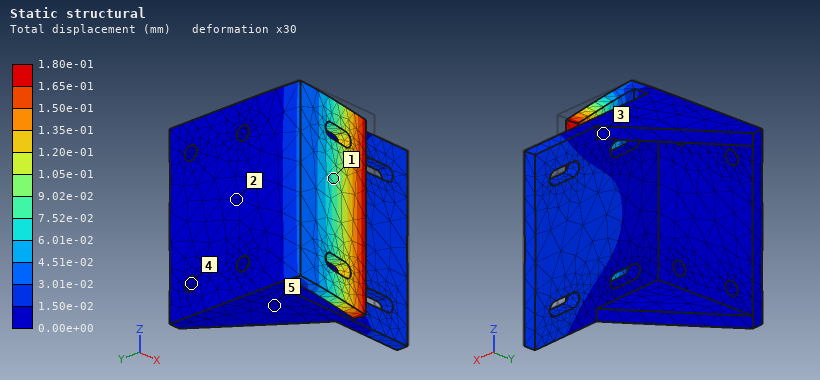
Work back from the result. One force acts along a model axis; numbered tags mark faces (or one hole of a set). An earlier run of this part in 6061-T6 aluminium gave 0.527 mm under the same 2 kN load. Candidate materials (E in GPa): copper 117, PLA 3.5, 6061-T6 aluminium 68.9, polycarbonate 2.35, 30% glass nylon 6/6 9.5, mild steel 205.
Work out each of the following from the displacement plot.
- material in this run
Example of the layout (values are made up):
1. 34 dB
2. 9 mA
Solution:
1. mild steel
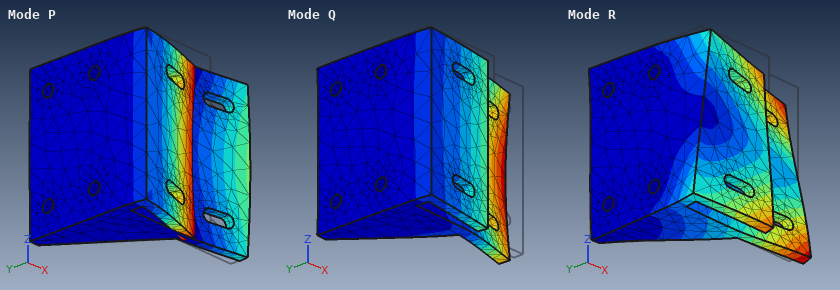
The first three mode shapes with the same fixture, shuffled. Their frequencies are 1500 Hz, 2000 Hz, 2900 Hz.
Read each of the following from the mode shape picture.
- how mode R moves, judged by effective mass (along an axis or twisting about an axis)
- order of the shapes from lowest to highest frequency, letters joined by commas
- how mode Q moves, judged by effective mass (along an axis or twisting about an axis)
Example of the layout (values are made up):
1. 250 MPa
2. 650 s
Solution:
1. along Z
2. Q, P, R
3. along Y
